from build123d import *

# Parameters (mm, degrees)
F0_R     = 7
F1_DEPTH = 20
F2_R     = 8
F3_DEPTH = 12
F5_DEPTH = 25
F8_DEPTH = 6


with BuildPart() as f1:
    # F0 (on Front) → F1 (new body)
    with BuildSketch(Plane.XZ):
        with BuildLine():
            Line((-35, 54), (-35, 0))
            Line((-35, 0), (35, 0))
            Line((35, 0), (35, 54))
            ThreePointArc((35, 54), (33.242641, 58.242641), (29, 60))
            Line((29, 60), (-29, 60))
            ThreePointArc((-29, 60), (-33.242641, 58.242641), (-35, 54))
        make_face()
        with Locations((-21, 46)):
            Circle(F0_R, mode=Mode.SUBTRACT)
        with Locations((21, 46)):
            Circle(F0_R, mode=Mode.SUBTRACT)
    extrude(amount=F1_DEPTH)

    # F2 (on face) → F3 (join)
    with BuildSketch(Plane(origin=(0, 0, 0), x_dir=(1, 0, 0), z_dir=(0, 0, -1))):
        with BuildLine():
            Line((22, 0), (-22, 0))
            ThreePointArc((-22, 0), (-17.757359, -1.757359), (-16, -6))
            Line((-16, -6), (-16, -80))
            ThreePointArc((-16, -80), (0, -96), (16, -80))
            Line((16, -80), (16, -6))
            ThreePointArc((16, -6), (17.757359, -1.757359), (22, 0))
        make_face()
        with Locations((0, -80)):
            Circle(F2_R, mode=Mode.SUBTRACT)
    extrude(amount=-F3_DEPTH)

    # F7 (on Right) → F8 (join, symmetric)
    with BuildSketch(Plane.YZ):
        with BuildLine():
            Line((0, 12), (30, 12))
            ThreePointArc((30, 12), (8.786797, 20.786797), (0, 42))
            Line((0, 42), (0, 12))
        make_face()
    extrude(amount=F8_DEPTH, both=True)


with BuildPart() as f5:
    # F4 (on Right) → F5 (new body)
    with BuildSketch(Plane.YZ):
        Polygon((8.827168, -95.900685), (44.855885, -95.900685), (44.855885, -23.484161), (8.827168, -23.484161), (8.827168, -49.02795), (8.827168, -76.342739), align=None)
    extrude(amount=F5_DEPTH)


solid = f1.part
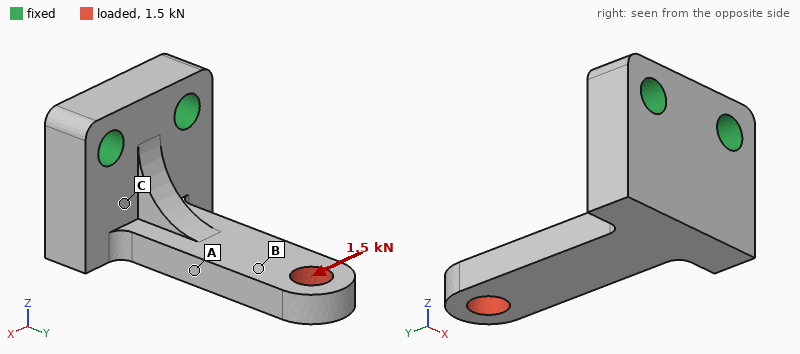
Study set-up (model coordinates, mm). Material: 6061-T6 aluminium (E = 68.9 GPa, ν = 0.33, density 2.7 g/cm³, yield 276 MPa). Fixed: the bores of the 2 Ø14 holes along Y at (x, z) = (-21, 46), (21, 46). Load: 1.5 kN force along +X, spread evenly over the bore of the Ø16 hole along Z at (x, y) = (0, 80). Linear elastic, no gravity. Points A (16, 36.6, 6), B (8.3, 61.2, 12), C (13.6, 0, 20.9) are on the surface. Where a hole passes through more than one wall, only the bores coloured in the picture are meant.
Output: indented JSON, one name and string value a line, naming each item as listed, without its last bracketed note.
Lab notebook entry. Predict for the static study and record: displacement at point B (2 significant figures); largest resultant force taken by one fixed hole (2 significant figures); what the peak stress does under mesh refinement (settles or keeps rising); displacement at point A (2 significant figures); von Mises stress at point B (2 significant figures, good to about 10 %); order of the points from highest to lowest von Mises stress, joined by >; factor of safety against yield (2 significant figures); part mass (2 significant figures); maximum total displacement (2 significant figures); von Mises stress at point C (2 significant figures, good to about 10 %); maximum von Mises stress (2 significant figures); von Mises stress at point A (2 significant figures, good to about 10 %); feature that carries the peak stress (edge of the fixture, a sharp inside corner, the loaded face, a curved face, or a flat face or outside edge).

{
  "displacement at point B": "0.15 mm",
  "largest resultant force taken by one fixed hole": "3.0 kN",
  "what the peak stress does under mesh refinement": "settles",
  "displacement at point A": "0.088 mm",
  "von Mises stress at point B": "8.5 MPa",
  "order of the points from highest to lowest von Mises stress, joined by >": "A > C > B",
  "factor of safety against yield": "2.7",
  "part mass": "310 g",
  "maximum total displacement": "0.27 mm",
  "von Mises stress at point C": "20 MPa",
  "maximum von Mises stress": "100 MPa",
  "von Mises stress at point A": "32 MPa",
  "feature that carries the peak stress": "a curved face"
}
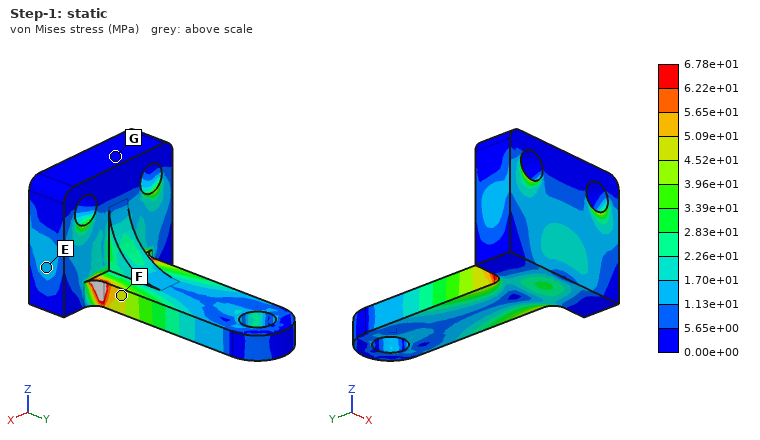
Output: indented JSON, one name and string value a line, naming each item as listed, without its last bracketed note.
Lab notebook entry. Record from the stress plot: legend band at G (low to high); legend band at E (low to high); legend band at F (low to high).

{
  "legend band at G": "0.00e+00 to 5.65e+00 MPa",
  "legend band at E": "1.13e+01 to 1.70e+01 MPa",
  "legend band at F": "4.52e+01 to 5.09e+01 MPa"
}
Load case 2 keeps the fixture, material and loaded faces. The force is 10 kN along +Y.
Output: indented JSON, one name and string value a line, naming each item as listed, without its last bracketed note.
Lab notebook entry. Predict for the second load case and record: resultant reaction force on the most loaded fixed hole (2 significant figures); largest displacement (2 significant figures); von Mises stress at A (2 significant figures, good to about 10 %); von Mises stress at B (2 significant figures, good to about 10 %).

{
  "resultant reaction force on the most loaded fixed hole": "5.0 kN",
  "largest displacement": "0.29 mm",
  "von Mises stress at A": "26 MPa",
  "von Mises stress at B": "26 MPa"
}
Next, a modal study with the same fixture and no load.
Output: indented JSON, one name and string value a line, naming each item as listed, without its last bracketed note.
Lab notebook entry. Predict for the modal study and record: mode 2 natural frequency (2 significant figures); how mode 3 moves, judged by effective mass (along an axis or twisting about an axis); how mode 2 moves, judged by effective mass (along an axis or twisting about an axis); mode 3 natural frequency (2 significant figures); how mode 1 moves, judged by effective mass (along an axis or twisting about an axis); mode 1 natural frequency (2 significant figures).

{
  "mode 2 natural frequency": "2300 Hz",
  "how mode 3 moves, judged by effective mass": "along Y",
  "how mode 2 moves, judged by effective mass": "along X",
  "mode 3 natural frequency": "4700 Hz",
  "how mode 1 moves, judged by effective mass": "along Z",
  "mode 1 natural frequency": "1300 Hz"
}
